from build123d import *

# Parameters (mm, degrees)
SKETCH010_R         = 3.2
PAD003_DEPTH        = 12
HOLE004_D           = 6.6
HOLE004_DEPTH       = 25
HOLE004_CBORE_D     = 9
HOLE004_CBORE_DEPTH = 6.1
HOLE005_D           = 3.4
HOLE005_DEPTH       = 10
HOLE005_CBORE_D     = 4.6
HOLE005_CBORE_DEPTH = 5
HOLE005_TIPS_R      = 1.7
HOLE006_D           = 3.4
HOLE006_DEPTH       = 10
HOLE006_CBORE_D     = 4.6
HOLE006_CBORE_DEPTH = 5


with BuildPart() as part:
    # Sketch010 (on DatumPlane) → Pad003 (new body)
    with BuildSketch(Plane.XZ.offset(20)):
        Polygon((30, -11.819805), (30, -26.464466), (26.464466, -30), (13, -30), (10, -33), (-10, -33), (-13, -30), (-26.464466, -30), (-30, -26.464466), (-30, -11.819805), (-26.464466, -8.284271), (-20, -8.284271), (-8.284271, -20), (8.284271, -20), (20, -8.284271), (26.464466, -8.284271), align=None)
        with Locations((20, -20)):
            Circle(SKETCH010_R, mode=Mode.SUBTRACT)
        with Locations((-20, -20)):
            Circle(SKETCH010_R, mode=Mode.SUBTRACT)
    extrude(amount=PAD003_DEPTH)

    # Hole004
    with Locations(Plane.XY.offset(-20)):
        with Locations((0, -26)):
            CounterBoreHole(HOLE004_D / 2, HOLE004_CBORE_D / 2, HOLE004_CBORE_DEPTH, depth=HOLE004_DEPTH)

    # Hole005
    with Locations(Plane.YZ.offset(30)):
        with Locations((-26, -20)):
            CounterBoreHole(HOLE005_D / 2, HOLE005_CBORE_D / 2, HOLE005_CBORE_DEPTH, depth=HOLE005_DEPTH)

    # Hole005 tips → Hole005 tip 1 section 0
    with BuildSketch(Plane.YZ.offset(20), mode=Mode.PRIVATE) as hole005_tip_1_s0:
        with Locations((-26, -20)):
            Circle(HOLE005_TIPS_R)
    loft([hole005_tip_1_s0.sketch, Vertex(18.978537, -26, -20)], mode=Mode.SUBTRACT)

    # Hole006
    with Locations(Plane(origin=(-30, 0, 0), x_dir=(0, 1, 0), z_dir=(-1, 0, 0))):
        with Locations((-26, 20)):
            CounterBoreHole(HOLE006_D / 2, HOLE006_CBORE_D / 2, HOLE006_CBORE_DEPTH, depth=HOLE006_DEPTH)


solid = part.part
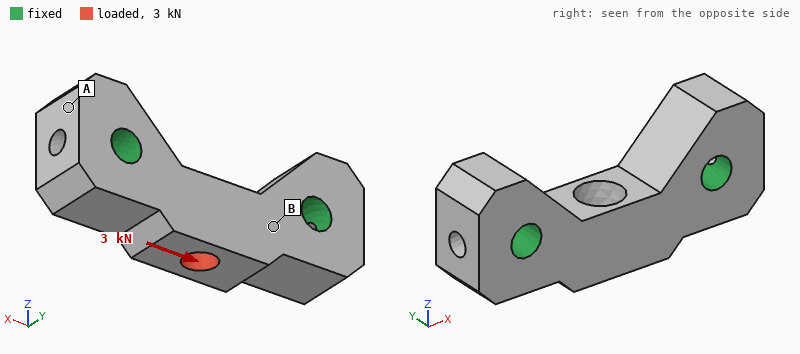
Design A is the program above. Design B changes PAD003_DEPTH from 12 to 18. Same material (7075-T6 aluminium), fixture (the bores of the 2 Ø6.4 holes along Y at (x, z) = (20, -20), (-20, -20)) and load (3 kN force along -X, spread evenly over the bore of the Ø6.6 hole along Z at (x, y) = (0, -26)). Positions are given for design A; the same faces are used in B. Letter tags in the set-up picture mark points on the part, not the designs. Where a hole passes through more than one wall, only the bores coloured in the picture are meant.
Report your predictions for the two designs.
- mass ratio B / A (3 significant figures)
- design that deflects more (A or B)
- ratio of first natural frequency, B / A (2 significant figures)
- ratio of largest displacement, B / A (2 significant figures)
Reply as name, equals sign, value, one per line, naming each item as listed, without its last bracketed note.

mass ratio B / A = 1.54
design that deflects more = A
ratio of first natural frequency, B / A = 1.1
ratio of largest displacement, B / A = 0.88
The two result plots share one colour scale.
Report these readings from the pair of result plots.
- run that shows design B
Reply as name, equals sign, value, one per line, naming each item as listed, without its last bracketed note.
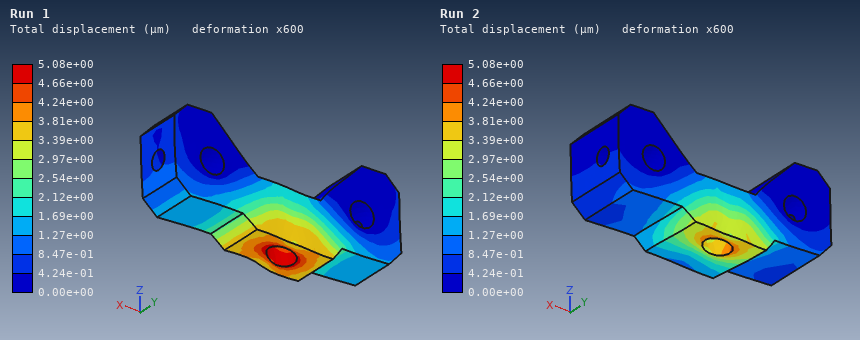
run that shows design B = Run 2
